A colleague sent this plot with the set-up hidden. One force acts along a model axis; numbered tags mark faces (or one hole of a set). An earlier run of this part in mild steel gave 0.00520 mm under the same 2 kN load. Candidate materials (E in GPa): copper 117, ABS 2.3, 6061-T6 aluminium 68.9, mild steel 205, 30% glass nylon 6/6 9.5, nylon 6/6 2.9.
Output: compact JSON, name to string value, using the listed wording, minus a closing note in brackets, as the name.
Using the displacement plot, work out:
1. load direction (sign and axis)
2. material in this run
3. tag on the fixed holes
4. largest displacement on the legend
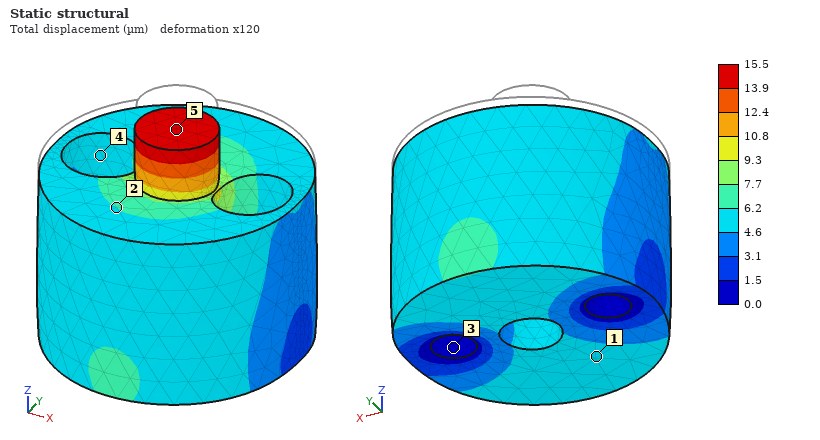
{"load direction": "-Z", "material in this run": "6061-T6 aluminium", "tag on the fixed holes": "3", "largest displacement on the legend": "15.5 µm"}
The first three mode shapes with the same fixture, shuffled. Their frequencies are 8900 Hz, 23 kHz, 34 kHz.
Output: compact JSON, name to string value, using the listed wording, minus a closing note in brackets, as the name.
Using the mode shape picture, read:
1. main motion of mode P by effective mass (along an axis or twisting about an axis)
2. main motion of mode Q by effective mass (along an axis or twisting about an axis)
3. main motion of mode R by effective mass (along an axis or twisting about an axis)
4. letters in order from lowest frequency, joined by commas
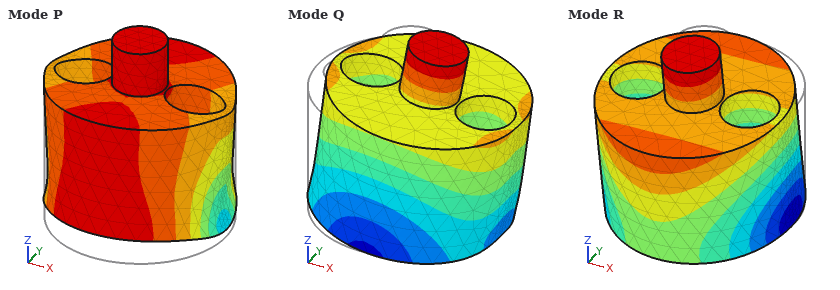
{"main motion of mode P by effective mass": "along Z", "main motion of mode Q by effective mass": "along X", "main motion of mode R by effective mass": "along Y", "letters in order from lowest frequency, joined by commas": "R, Q, P"}
